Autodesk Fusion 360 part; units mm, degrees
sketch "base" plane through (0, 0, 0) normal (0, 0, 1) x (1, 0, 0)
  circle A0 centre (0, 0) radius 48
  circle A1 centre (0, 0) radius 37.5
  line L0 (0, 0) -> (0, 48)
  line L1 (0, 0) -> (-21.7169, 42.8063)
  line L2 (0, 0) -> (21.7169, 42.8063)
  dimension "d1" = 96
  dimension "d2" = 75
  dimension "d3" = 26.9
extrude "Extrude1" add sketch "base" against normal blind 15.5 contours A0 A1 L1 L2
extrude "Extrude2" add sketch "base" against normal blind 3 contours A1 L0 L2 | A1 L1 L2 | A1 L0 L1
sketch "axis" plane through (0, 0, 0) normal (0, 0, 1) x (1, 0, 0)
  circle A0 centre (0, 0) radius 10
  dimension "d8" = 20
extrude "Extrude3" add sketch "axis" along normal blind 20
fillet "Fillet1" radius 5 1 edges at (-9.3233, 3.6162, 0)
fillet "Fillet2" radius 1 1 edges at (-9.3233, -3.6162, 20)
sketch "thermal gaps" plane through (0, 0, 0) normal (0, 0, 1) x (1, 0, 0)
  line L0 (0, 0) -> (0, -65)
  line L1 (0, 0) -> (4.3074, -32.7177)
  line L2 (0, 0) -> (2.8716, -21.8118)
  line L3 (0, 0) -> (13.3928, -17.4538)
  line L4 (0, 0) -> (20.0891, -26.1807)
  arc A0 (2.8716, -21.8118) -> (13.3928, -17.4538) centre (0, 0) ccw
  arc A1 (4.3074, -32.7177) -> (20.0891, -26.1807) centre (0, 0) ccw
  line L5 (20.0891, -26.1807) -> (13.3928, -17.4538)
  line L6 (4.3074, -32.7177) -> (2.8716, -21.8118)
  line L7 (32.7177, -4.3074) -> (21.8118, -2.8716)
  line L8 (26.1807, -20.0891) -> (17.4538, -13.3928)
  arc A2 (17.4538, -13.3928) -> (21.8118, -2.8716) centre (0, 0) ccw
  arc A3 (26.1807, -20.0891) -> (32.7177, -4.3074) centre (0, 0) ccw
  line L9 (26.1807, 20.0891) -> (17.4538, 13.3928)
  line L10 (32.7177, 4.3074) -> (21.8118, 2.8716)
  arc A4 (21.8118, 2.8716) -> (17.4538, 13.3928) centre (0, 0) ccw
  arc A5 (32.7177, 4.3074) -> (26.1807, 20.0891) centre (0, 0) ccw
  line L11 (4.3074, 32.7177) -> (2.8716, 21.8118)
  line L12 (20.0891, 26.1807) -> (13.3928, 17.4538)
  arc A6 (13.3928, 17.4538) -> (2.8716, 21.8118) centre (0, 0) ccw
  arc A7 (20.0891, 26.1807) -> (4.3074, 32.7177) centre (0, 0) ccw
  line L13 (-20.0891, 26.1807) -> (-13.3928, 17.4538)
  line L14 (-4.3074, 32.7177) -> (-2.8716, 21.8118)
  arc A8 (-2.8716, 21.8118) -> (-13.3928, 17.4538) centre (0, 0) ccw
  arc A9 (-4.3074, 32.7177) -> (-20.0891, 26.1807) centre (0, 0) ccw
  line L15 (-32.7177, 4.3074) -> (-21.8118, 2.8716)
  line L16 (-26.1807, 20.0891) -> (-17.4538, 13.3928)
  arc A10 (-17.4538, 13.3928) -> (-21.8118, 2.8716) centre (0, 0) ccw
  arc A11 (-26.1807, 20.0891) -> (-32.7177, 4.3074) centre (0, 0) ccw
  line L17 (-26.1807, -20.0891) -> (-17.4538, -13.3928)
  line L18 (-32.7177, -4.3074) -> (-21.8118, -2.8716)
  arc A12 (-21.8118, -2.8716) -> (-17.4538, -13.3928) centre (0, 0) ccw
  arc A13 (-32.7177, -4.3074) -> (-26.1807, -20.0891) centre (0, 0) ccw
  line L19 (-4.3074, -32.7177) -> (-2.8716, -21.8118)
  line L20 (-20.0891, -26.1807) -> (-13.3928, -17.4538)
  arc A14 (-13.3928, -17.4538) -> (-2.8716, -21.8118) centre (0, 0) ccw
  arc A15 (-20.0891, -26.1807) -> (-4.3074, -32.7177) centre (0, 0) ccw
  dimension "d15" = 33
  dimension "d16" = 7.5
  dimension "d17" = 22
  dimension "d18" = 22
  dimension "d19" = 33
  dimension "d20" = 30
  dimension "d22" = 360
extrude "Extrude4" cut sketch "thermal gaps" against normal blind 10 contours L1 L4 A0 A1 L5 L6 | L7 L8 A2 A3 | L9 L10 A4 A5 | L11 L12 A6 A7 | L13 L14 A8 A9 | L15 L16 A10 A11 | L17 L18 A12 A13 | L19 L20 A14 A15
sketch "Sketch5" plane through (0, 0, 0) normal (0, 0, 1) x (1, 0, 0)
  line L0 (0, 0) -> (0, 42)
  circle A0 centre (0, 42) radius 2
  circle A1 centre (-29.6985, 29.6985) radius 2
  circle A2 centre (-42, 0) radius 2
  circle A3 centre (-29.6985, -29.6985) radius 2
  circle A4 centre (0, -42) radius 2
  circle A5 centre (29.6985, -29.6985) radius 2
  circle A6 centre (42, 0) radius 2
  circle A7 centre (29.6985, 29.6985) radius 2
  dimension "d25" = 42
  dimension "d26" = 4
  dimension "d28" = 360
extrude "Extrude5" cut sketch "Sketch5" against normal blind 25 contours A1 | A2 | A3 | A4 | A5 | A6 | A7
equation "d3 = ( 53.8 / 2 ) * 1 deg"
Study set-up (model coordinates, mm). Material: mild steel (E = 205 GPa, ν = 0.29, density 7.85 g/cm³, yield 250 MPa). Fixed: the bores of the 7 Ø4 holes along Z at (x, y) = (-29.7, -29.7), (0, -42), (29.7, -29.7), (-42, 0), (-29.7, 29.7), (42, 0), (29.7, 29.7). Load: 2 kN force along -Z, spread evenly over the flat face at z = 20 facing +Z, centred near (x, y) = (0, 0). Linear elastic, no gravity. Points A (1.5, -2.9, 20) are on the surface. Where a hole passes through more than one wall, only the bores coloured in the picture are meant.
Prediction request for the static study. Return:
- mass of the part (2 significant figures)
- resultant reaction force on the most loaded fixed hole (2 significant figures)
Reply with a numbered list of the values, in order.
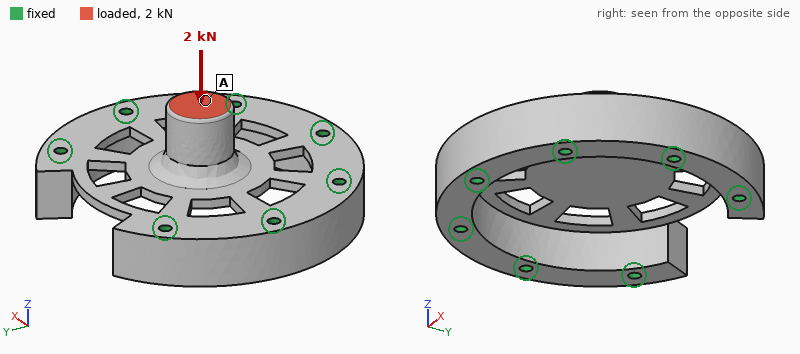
1. 410 g
2. 450 N
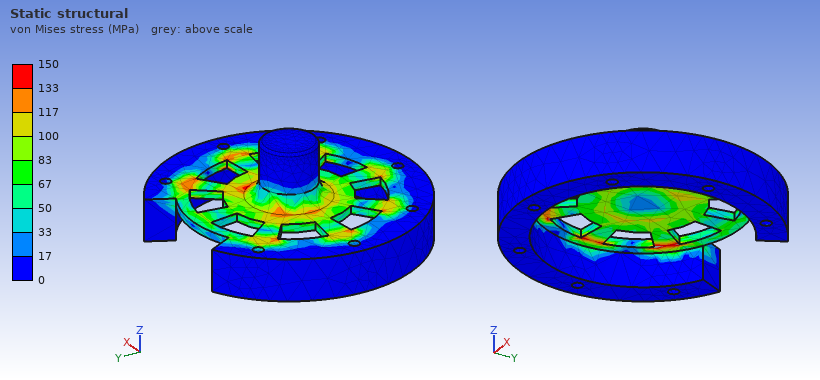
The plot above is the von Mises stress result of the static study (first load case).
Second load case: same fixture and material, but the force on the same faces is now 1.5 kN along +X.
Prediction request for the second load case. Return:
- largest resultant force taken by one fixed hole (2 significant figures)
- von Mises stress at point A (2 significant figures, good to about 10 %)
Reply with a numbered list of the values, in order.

1. 450 N
2. 10 MPa
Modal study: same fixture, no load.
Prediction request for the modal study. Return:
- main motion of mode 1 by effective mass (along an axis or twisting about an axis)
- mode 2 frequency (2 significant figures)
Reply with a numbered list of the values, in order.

1. along Z
2. 4300 Hz
